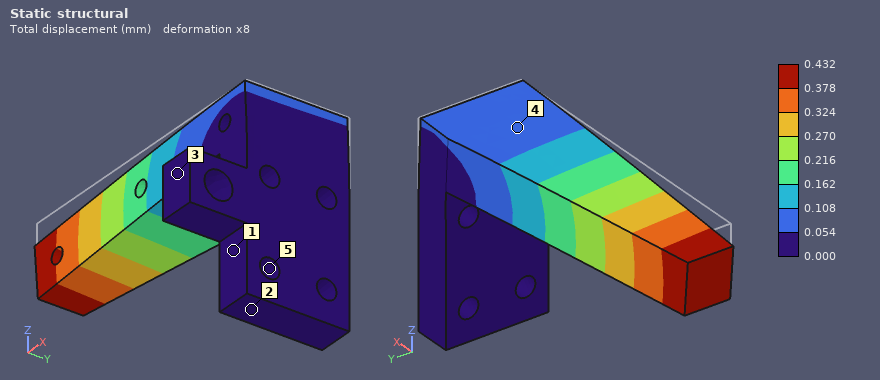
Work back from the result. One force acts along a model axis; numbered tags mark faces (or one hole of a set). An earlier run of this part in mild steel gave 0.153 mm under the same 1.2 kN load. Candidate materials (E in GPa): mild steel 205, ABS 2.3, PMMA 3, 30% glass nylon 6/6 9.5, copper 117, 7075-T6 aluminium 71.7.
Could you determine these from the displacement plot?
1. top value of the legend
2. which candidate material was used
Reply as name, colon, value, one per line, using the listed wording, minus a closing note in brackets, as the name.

top value of the legend: 0.432 mm
which candidate material was used: 7075-T6 aluminium
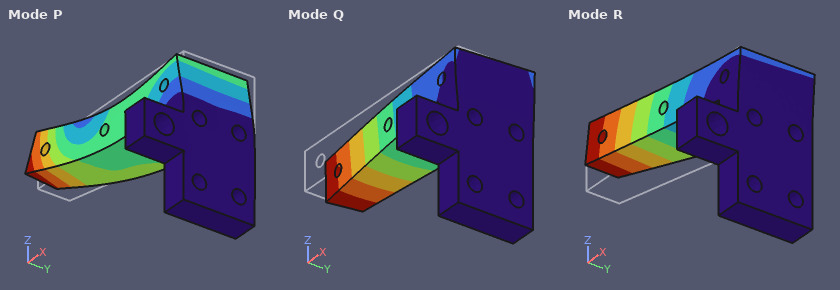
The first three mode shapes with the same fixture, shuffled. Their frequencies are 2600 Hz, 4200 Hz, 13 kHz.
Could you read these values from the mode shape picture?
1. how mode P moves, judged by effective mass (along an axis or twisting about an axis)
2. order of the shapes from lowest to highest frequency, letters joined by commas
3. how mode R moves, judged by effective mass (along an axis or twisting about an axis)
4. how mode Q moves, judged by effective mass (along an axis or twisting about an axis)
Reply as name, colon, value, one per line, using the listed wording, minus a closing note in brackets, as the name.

how mode P moves, judged by effective mass: along X
order of the shapes from lowest to highest frequency, letters joined by commas: R, Q, P
how mode R moves, judged by effective mass: along Z
how mode Q moves, judged by effective mass: along Y
